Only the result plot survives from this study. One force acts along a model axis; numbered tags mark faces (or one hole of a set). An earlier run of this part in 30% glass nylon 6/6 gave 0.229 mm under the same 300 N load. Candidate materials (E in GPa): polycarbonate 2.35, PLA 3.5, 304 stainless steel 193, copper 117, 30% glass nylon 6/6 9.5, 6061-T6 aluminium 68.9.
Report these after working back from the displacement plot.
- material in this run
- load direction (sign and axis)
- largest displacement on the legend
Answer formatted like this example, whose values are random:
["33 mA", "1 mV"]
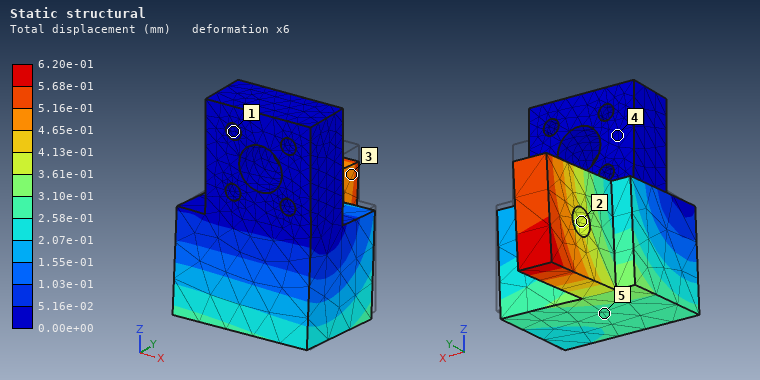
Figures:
["PLA", "-Z", "6.20e-01 mm"]
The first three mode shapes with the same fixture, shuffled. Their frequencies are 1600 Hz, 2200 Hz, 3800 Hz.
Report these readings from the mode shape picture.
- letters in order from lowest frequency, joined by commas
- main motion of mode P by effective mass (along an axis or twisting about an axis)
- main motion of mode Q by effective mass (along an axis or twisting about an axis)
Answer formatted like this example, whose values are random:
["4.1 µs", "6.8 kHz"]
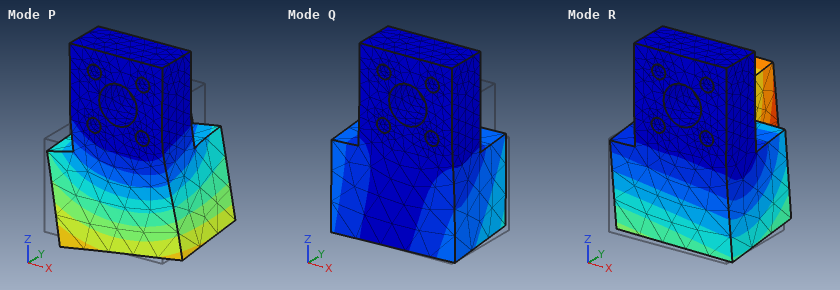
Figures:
["R, Q, P", "along X", "along X"]
